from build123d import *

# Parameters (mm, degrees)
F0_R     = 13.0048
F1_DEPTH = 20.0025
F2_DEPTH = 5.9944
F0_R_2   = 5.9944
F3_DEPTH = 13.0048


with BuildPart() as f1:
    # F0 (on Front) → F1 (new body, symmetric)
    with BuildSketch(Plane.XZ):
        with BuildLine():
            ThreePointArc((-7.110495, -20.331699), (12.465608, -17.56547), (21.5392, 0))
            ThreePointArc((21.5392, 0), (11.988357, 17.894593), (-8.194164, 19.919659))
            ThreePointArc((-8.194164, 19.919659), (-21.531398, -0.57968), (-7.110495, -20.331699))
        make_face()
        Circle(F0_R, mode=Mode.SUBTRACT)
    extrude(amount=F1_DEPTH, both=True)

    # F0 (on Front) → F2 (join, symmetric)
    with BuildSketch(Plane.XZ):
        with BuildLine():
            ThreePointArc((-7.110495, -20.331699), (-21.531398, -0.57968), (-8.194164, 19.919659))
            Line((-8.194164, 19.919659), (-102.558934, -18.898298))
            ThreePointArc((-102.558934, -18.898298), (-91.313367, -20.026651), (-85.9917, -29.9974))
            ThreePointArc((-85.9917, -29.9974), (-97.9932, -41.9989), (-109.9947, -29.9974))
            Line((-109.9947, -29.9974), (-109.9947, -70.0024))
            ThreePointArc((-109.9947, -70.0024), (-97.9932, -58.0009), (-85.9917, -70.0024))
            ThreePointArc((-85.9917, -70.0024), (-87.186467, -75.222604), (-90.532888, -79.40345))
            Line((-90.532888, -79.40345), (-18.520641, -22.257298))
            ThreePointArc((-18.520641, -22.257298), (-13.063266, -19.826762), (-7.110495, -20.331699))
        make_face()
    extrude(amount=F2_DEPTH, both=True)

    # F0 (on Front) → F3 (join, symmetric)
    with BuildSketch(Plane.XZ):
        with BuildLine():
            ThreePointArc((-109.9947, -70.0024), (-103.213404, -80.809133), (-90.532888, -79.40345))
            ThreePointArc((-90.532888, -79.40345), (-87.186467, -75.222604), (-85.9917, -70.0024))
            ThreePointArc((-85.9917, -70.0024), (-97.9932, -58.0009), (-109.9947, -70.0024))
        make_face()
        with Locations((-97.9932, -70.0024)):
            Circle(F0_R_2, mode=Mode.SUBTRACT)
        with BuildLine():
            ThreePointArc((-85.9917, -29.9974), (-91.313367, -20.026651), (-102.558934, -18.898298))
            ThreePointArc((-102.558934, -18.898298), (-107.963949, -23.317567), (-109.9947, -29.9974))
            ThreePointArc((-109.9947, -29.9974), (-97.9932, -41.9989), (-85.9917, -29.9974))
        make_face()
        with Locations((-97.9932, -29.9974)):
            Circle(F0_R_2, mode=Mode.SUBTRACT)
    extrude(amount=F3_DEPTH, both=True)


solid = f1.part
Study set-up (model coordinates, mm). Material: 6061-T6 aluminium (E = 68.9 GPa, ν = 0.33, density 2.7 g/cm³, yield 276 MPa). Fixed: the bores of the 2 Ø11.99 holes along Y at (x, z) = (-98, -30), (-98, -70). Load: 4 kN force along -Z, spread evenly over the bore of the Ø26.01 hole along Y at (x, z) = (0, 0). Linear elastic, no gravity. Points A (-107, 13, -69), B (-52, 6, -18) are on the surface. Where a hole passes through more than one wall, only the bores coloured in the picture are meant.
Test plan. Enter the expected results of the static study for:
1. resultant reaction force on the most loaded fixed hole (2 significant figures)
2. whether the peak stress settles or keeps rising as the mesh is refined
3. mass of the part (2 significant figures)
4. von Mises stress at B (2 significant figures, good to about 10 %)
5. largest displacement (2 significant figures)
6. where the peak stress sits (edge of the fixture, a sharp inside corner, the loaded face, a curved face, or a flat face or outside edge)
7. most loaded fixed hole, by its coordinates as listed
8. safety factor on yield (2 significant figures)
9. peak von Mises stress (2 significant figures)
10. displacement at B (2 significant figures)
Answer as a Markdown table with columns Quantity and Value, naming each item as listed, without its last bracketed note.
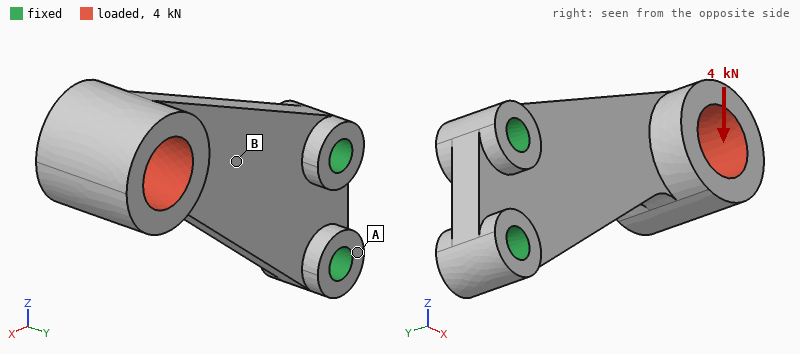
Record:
| Quantity | Value |
|---|---|
| resultant reaction force on the most loaded fixed hole | 9.4 kN |
| whether the peak stress settles or keeps rising as the mesh is refined | settles |
| mass of the part | 280 g |
| von Mises stress at B | 11 MPa |
| largest displacement | 0.29 mm |
| where the peak stress sits | a curved face |
| most loaded fixed hole, by its coordinates as listed | (-98, -70) |
| safety factor on yield | 4.1 |
| peak von Mises stress | 68 MPa |
| displacement at B | 0.049 mm |
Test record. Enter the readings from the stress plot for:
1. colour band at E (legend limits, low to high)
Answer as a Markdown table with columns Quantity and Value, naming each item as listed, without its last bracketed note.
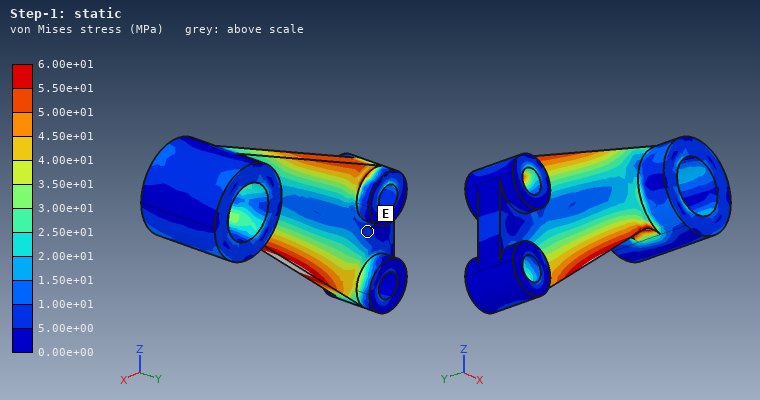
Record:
| Quantity | Value |
|---|---|
| colour band at E | 5.00e+00 to 1.00e+01 MPa |
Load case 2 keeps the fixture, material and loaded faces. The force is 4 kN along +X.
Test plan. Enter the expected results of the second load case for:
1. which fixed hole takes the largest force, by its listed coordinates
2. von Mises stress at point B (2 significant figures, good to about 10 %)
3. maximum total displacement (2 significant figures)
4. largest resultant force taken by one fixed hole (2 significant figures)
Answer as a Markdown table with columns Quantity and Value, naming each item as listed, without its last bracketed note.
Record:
| Quantity | Value |
|---|---|
| which fixed hole takes the largest force, by its listed coordinates | (-98, -30) |
| von Mises stress at point B | 12 MPa |
| maximum total displacement | 0.11 mm |
| largest resultant force taken by one fixed hole | 6.4 kN |
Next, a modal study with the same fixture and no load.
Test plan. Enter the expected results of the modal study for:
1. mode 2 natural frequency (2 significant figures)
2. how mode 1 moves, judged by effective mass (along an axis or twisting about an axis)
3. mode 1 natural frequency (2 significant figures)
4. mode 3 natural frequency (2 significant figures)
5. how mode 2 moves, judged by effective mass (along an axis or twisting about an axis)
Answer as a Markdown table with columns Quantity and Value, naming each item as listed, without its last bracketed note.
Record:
| Quantity | Value |
|---|---|
| mode 2 natural frequency | 1900 Hz |
| how mode 1 moves, judged by effective mass | along Y |
| mode 1 natural frequency | 570 Hz |
| mode 3 natural frequency | 2300 Hz |
| how mode 2 moves, judged by effective mass | along Z |
